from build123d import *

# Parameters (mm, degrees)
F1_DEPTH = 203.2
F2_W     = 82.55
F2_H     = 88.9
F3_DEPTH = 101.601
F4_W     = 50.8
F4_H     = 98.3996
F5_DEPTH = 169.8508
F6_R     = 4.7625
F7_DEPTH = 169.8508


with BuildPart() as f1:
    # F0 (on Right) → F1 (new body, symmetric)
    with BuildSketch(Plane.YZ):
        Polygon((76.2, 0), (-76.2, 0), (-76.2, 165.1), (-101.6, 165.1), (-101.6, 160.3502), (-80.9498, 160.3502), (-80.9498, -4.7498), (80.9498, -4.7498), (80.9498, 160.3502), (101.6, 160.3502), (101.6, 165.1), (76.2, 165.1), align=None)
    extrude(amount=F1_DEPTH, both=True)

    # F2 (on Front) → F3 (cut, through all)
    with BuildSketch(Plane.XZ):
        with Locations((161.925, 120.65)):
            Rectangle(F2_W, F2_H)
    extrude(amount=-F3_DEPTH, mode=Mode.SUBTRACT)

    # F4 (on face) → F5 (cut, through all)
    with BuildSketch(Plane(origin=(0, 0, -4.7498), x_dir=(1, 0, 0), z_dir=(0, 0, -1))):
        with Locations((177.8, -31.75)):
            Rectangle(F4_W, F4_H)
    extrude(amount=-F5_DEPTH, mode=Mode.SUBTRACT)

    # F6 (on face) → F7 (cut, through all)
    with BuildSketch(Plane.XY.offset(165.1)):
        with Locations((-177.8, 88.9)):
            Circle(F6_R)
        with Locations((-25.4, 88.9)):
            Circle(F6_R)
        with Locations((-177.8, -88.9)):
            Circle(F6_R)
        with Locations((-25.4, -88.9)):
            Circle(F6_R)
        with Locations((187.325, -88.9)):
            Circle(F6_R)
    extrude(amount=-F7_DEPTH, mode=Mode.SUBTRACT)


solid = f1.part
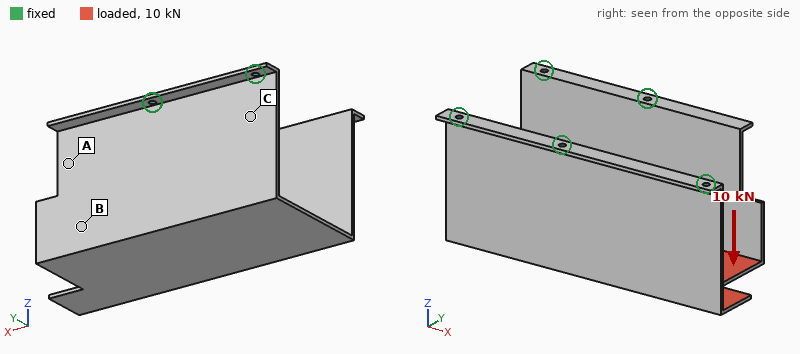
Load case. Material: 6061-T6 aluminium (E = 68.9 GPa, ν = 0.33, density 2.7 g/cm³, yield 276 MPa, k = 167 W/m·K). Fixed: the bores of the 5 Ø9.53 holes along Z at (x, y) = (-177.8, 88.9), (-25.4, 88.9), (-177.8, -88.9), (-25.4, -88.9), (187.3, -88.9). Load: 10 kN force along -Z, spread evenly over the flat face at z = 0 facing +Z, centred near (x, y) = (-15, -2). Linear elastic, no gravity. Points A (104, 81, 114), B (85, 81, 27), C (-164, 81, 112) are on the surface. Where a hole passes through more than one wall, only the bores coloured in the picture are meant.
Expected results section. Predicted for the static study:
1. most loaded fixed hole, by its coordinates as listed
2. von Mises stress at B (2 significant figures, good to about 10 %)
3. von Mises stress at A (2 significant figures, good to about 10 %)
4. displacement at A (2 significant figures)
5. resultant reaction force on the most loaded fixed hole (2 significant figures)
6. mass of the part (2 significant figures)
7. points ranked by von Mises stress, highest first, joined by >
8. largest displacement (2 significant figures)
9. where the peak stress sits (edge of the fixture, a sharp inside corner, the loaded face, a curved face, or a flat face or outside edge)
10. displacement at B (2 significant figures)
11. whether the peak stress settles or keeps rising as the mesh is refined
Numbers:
(-25.4, 88.9)
39 MPa
17 MPa
0.54 mm
4.6 kN
2.5 kg
B > A > C
1.4 mm
edge of the fixture
0.56 mm
keeps rising
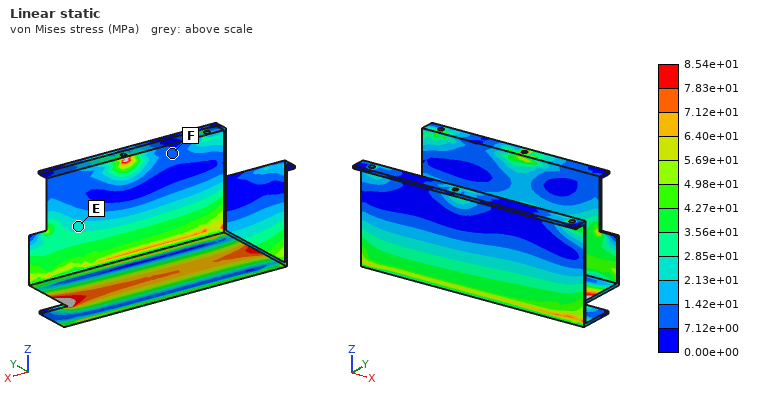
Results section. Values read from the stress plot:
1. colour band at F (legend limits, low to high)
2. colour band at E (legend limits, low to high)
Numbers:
7.12e+00 to 1.42e+01 MPa
2.13e+01 to 2.85e+01 MPa
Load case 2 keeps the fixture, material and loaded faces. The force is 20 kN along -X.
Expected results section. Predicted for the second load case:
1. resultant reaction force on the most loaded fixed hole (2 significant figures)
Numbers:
11 kN
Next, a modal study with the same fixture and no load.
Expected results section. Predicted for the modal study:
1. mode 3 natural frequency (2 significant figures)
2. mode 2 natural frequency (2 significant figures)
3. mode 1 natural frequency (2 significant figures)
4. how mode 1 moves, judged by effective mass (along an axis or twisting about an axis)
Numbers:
510 Hz
460 Hz
110 Hz
along Y
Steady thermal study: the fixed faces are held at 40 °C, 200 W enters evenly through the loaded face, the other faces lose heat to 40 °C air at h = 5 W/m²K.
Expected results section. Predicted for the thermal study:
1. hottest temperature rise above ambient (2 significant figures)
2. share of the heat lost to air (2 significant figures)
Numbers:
72 K
35 %
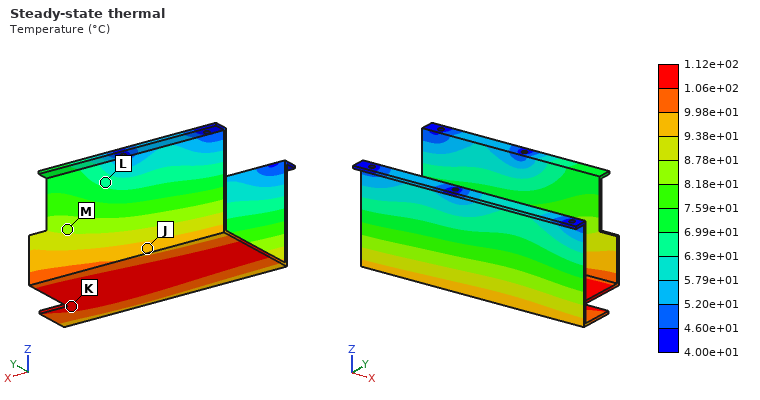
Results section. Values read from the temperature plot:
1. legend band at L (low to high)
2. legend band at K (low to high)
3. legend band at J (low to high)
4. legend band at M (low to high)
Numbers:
6.39e+01 to 6.99e+01 °C
1.06e+02 to 1.12e+02 °C
9.38e+01 to 9.98e+01 °C
8.18e+01 to 8.78e+01 °C
